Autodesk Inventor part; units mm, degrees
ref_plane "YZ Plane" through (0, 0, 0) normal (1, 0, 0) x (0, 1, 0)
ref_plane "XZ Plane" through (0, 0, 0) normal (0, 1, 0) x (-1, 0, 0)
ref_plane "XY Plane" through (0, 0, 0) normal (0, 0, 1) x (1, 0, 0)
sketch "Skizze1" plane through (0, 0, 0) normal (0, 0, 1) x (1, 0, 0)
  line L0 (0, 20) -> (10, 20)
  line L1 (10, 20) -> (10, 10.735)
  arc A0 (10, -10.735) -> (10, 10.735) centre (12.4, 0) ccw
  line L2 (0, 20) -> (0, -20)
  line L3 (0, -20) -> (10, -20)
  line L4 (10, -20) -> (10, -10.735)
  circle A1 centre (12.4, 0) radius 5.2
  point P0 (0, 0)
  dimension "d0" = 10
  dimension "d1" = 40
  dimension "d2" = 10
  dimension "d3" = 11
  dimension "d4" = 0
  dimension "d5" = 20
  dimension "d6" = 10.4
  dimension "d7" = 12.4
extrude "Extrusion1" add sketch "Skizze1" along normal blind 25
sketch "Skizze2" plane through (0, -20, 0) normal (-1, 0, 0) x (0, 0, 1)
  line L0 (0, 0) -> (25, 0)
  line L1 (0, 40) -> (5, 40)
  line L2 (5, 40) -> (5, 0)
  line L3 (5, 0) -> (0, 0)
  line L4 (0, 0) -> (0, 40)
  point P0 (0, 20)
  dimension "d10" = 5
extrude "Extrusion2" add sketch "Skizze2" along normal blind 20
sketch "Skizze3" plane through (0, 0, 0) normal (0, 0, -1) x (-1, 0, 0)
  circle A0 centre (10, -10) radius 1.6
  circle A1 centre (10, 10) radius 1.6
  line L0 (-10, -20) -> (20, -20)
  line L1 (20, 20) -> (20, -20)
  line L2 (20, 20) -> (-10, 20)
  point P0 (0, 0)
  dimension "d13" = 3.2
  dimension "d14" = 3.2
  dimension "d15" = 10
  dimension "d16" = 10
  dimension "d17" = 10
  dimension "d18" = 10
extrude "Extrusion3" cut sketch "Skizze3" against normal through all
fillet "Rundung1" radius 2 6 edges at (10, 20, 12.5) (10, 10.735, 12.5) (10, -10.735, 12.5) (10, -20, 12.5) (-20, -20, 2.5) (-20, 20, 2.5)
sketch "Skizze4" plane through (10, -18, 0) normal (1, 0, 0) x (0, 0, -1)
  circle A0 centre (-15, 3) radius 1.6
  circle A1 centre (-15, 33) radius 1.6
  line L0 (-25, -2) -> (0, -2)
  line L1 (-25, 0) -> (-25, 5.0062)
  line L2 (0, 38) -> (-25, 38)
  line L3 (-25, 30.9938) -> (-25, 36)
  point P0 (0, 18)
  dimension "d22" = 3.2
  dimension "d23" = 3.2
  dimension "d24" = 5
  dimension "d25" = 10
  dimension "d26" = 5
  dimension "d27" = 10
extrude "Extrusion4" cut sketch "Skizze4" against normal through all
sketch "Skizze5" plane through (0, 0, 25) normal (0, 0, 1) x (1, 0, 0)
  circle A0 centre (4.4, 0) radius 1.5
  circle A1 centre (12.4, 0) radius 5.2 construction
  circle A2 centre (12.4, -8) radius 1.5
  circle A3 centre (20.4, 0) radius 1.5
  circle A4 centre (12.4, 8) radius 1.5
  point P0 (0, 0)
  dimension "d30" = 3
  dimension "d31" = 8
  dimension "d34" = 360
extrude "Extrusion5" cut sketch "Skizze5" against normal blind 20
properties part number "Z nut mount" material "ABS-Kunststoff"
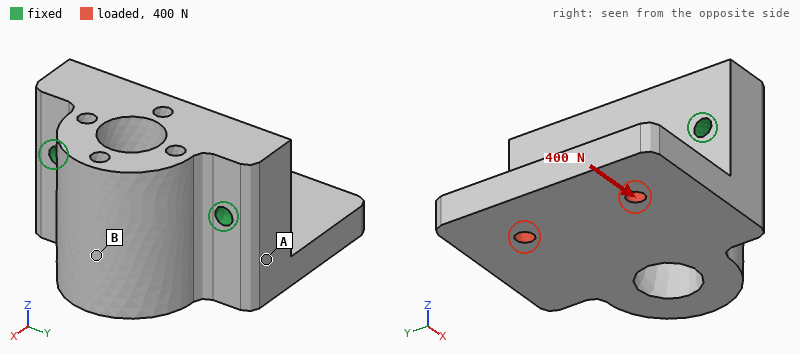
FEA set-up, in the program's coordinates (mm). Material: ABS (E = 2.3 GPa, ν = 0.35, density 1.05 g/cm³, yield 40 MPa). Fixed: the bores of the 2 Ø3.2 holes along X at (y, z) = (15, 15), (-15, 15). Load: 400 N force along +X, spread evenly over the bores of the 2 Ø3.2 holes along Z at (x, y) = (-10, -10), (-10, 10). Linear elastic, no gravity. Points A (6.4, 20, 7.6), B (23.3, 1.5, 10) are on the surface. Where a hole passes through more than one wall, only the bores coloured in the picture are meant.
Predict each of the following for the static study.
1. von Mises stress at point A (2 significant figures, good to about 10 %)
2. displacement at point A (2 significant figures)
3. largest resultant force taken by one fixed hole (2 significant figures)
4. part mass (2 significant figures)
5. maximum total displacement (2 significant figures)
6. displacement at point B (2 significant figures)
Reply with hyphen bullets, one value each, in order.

- 3.9 MPa
- 0.033 mm
- 200 N
- 18 g
- 0.19 mm
- 0.087 mm
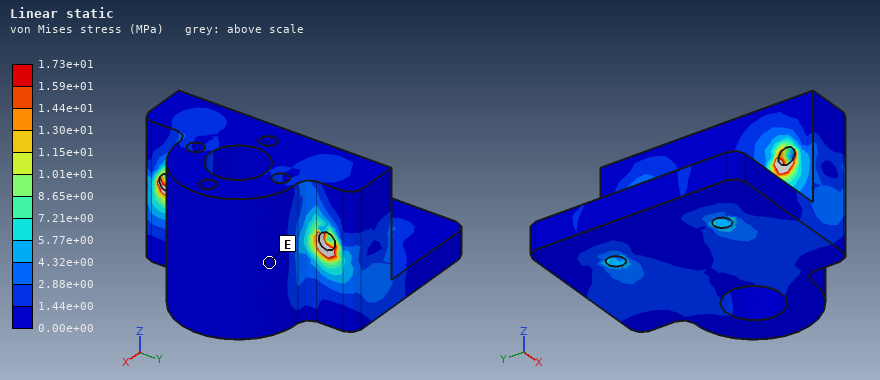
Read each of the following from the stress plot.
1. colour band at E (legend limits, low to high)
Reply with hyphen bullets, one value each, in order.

- 0.00e+00 to 1.44e+00 MPa
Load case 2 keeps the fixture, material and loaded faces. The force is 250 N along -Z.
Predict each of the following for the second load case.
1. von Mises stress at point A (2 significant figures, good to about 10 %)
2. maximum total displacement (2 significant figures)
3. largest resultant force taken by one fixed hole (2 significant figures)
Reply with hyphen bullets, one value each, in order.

- 2.8 MPa
- 0.54 mm
- 130 N
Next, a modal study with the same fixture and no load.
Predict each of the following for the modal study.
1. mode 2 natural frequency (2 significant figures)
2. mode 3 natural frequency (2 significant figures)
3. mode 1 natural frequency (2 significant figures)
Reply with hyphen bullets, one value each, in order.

- 3300 Hz
- 3900 Hz
- 1900 Hz
